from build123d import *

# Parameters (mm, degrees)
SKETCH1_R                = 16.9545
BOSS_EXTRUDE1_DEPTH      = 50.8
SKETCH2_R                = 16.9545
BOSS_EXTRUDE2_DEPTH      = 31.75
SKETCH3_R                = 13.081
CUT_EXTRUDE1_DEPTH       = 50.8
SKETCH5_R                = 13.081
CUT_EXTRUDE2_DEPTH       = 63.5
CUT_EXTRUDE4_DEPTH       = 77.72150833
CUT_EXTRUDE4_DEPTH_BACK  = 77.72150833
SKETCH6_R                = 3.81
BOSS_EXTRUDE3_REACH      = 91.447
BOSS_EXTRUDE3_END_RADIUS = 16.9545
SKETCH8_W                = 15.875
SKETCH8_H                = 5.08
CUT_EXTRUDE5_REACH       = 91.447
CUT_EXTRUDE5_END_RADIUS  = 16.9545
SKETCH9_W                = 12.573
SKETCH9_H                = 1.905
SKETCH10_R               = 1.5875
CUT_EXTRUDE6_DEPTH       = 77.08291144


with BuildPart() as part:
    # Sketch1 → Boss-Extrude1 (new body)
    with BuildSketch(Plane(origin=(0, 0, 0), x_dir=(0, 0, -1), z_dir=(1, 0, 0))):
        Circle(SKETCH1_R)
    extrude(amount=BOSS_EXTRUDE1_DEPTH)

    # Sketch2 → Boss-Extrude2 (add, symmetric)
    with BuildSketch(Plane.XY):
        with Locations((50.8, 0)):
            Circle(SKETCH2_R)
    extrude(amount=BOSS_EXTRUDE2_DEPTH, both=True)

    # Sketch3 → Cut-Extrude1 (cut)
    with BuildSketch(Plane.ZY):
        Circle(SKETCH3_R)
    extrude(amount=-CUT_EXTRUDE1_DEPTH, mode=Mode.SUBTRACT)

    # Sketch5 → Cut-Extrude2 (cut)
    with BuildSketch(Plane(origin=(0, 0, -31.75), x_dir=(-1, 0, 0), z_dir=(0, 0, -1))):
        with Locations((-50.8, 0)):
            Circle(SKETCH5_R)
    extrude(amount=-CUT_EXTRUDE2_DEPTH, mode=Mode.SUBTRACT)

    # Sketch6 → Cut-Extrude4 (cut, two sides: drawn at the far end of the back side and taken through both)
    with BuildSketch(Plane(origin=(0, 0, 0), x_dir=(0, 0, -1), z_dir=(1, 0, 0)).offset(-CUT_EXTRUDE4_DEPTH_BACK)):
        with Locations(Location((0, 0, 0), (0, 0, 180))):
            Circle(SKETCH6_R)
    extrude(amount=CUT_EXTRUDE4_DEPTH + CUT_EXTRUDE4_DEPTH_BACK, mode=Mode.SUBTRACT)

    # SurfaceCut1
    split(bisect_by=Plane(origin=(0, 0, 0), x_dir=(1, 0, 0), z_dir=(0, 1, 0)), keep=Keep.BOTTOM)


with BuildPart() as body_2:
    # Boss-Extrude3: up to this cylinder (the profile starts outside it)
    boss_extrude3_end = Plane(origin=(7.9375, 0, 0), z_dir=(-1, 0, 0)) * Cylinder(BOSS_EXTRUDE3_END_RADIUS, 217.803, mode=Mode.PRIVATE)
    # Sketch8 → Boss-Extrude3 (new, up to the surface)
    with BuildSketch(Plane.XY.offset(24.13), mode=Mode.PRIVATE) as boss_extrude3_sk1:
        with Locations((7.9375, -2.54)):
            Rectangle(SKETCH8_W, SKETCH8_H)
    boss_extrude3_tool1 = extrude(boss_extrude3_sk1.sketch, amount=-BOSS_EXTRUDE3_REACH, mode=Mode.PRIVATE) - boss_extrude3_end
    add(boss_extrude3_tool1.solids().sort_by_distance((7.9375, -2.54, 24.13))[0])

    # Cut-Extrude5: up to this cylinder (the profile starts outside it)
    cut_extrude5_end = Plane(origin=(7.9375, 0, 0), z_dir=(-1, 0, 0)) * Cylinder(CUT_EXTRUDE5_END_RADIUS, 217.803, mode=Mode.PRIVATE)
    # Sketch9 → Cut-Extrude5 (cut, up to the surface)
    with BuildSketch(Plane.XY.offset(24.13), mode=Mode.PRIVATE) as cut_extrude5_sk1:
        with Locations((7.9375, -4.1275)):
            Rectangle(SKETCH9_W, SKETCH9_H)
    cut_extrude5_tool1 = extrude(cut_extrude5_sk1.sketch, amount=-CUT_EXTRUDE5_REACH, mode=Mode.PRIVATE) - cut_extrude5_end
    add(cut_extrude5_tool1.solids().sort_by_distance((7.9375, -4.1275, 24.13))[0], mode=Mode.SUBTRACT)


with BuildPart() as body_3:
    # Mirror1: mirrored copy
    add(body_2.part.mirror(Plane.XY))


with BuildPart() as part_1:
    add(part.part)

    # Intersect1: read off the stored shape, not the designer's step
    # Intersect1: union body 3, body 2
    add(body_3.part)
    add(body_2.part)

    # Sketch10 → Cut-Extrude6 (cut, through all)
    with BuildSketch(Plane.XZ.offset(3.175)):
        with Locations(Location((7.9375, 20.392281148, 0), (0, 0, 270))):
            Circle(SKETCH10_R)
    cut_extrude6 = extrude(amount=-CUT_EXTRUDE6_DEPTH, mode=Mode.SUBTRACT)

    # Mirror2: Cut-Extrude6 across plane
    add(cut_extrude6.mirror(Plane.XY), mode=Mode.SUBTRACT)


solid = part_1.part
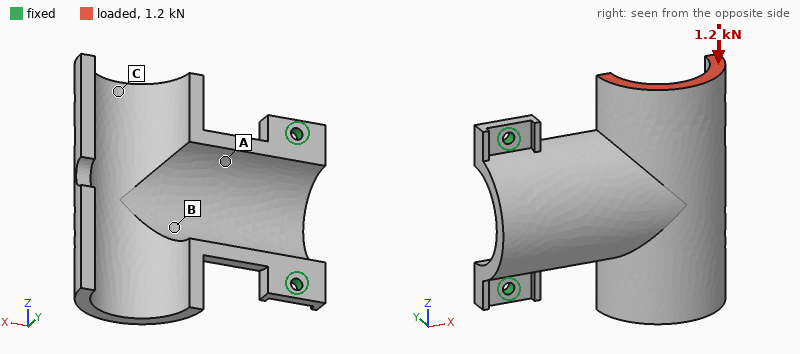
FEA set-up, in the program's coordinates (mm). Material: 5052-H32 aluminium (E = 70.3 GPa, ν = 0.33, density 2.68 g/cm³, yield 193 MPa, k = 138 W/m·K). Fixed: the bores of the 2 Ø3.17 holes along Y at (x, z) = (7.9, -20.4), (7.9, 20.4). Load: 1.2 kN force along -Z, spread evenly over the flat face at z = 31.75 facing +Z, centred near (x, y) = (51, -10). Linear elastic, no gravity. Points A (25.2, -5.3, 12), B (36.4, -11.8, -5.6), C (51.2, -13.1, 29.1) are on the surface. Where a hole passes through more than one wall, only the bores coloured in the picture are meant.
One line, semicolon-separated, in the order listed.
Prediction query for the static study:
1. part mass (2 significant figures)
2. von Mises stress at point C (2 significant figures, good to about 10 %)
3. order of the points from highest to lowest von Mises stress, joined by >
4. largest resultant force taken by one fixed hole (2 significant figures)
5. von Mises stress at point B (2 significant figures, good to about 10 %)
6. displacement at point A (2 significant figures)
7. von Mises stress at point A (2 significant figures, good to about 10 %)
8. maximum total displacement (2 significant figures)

48 g; 18 MPa; A > B > C; 1.4 kN; 57 MPa; 0.076 mm; 99 MPa; 0.44 mm
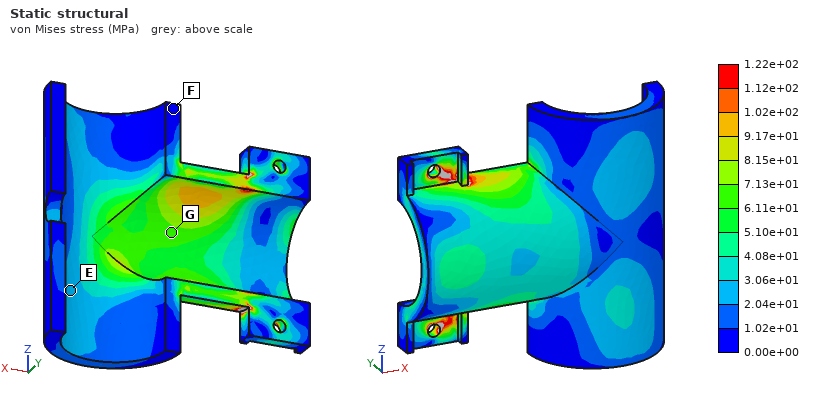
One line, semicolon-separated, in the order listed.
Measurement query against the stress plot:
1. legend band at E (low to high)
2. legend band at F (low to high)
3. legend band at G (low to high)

2.04e+01 to 3.06e+01 MPa; 0.00e+00 to 1.02e+01 MPa; 6.11e+01 to 7.13e+01 MPa
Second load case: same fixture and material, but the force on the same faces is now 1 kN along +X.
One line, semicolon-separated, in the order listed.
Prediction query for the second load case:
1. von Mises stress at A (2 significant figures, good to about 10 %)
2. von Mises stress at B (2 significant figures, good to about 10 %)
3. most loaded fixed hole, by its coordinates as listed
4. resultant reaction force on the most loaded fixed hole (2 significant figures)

51 MPa; 34 MPa; (7.9, 20.4); 1.3 kN
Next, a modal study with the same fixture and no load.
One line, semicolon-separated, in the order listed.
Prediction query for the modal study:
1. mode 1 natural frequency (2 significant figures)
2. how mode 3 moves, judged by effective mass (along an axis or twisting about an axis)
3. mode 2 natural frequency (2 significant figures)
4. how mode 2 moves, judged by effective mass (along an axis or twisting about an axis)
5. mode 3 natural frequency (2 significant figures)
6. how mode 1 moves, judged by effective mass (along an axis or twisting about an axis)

810 Hz; along Z; 1500 Hz; along Z; 3700 Hz; along Y
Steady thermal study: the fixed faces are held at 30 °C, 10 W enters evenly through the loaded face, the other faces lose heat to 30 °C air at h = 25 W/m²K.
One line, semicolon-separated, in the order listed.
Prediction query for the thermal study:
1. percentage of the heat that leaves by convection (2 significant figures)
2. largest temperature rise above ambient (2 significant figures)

30 %; 25 K
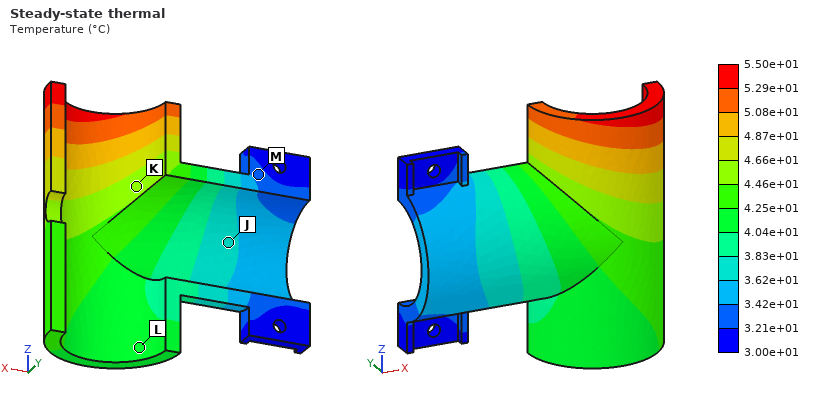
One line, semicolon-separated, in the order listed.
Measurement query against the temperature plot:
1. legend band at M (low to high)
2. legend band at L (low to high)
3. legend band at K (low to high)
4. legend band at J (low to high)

3.21e+01 to 3.42e+01 °C; 4.04e+01 to 4.25e+01 °C; 4.46e+01 to 4.66e+01 °C; 3.62e+01 to 3.83e+01 °C
